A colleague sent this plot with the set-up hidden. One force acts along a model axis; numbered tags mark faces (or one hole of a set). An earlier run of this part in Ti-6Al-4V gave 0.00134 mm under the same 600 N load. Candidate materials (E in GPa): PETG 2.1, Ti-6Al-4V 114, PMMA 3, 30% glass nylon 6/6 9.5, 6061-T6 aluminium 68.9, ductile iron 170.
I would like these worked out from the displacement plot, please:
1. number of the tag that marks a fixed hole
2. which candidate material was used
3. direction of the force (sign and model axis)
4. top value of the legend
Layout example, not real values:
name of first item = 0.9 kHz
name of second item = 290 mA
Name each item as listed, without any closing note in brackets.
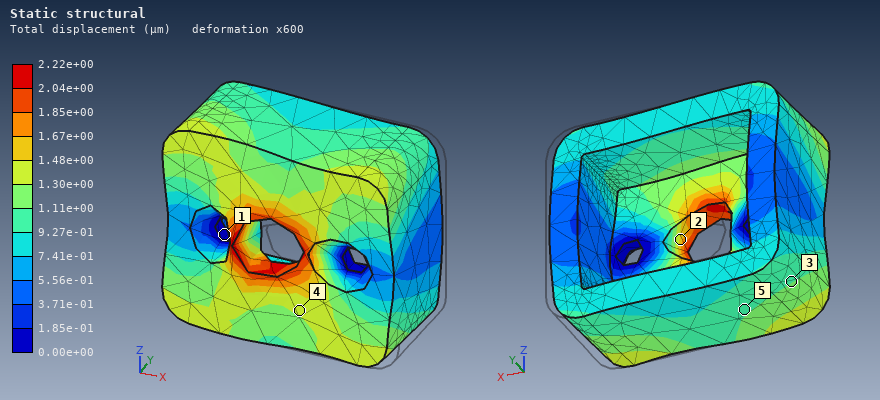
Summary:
number of the tag that marks a fixed hole = 1
which candidate material was used = 6061-T6 aluminium
direction of the force = -X
top value of the legend = 2.22e+00 µm
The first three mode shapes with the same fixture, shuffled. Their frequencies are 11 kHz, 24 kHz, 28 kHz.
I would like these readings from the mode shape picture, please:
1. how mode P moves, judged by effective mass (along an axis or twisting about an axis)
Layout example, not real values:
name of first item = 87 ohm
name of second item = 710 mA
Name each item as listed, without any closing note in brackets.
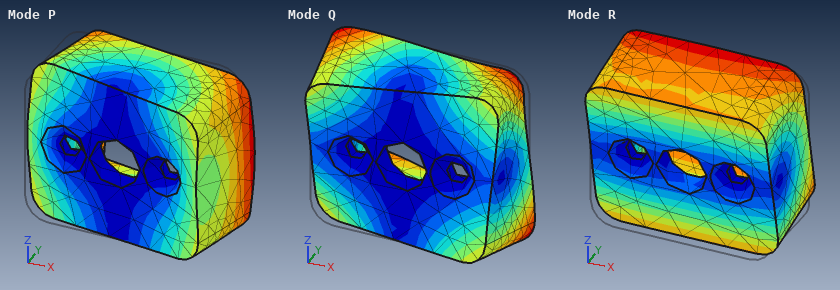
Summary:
how mode P moves, judged by effective mass = along X
